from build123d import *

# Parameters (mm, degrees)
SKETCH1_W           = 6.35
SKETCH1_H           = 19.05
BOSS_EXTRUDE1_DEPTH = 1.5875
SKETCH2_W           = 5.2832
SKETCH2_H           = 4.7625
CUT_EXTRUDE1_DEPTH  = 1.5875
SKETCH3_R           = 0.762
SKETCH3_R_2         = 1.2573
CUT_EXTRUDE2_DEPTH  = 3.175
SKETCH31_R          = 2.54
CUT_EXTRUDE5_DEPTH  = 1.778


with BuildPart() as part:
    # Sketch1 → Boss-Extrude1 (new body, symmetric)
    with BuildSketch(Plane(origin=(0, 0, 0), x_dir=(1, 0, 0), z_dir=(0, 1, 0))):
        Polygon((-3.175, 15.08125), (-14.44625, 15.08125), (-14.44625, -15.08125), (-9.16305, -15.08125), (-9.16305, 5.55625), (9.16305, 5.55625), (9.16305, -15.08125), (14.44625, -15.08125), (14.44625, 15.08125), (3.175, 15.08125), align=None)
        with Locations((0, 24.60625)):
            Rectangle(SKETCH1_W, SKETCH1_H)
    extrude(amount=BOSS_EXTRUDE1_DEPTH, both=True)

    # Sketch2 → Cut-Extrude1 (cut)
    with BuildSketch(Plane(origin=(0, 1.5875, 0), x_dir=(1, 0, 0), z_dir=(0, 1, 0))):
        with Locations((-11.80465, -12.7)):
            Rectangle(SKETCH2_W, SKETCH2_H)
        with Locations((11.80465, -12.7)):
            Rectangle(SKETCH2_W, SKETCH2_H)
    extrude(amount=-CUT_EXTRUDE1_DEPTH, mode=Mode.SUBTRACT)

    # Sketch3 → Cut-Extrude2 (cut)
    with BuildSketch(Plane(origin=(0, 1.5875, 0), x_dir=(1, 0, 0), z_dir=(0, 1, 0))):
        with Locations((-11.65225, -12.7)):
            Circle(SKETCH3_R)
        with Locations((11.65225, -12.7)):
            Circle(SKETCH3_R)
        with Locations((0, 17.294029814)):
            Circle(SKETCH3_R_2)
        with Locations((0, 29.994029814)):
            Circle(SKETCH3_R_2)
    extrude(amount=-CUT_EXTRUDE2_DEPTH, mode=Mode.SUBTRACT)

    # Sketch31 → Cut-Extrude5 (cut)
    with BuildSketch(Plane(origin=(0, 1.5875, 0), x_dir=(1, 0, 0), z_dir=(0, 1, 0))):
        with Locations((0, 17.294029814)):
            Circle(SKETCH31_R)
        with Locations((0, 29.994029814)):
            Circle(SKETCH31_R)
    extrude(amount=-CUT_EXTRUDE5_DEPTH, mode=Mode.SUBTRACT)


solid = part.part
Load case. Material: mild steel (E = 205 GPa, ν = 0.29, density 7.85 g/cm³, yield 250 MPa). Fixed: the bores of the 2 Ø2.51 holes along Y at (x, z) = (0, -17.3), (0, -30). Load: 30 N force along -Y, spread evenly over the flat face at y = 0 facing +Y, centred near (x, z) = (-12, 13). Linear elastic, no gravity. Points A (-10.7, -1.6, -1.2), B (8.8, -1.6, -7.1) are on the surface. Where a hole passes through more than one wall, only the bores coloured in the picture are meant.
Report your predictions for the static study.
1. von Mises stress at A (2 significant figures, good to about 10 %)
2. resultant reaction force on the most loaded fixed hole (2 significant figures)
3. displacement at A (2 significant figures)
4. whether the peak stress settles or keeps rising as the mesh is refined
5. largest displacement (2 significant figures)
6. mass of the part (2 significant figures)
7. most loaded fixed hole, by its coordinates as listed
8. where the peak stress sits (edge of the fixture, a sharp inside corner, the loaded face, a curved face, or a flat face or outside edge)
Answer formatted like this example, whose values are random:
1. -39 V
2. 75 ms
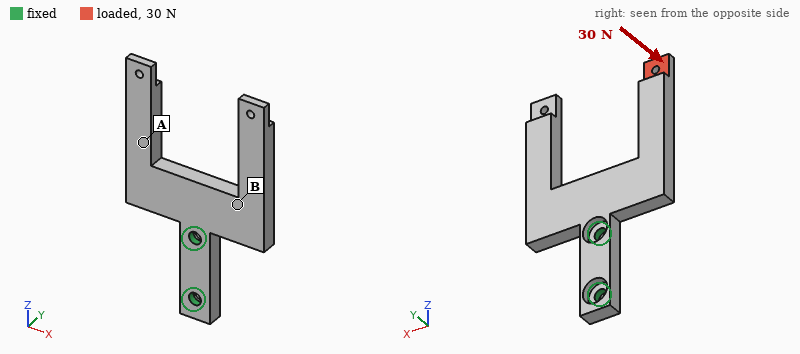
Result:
1. 47 MPa
2. 110 N
3. 0.060 mm
4. keeps rising
5. 0.15 mm
6. 14 g
7. (0, -17.3)
8. edge of the fixture
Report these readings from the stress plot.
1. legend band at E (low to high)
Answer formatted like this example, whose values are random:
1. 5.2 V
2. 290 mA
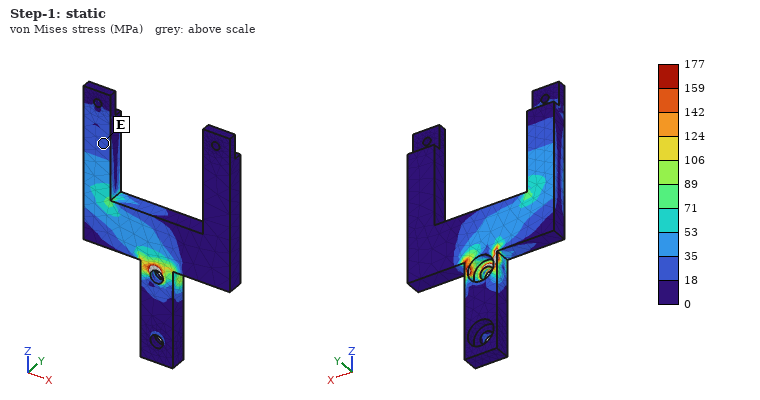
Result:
1. 18 to 35 MPa
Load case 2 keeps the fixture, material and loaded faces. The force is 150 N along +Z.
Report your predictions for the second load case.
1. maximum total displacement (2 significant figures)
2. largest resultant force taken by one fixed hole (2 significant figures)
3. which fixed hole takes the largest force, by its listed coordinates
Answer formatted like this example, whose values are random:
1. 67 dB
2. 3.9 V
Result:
1. 45 µm
2. 150 N
3. (0, -17.3)
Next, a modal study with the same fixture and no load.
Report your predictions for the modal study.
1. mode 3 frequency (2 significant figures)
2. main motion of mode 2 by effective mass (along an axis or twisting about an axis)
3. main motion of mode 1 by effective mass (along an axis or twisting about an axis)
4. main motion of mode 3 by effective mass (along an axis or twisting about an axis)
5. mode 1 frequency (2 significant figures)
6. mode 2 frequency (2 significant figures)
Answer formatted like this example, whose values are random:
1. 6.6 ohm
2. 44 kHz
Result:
1. 3300 Hz
2. twisting about Z
3. along Y
4. along X
5. 1900 Hz
6. 2400 Hz
